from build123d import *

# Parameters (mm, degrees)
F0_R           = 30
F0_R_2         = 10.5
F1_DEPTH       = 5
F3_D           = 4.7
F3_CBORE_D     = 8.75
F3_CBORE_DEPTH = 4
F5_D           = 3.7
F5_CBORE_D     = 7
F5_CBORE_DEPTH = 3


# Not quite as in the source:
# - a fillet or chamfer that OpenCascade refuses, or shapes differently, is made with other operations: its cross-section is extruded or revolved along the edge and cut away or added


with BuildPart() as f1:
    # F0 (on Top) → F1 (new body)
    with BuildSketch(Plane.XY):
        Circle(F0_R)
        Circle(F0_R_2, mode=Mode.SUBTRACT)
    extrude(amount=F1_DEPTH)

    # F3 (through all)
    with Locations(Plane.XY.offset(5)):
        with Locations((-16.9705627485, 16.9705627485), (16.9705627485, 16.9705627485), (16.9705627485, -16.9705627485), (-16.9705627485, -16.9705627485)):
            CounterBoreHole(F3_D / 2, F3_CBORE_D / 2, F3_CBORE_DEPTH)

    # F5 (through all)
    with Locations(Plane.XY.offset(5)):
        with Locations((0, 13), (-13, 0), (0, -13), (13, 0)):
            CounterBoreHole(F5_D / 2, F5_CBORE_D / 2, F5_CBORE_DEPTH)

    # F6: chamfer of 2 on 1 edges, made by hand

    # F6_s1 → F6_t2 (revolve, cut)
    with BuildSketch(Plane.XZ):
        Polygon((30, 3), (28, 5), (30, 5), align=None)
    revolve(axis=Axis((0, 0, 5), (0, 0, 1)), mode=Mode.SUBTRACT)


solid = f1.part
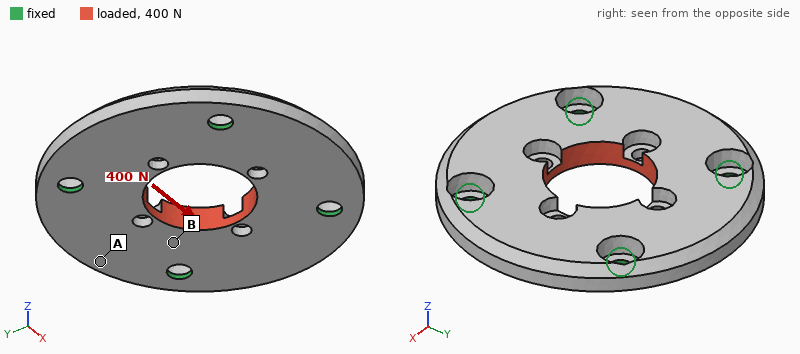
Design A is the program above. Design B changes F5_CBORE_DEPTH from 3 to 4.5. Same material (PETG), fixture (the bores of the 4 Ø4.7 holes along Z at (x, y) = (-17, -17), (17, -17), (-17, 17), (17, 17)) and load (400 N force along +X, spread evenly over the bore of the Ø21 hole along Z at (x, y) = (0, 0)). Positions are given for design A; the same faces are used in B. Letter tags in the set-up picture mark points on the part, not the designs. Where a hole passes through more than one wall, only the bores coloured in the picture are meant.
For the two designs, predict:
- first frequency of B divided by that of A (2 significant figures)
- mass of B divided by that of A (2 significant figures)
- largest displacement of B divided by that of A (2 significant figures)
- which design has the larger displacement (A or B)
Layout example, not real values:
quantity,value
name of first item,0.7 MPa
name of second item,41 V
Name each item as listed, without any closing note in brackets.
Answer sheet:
quantity,value
first frequency of B divided by that of A,0.99
mass of B divided by that of A,0.99
largest displacement of B divided by that of A,1.1
which design has the larger displacement,B
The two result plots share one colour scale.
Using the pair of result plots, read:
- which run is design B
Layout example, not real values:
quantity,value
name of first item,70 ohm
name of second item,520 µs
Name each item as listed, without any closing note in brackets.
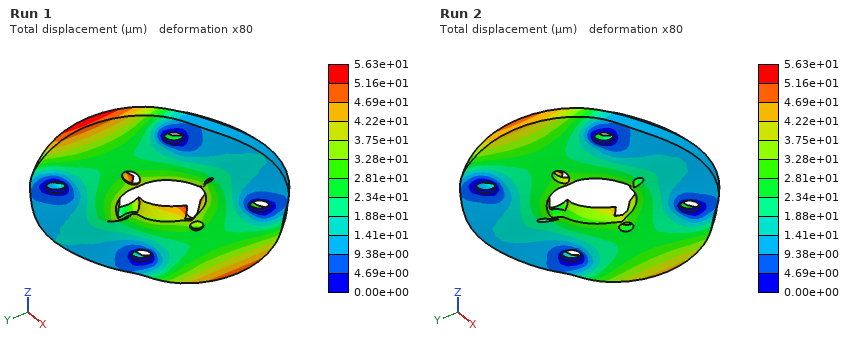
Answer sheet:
quantity,value
which run is design B,Run 1
